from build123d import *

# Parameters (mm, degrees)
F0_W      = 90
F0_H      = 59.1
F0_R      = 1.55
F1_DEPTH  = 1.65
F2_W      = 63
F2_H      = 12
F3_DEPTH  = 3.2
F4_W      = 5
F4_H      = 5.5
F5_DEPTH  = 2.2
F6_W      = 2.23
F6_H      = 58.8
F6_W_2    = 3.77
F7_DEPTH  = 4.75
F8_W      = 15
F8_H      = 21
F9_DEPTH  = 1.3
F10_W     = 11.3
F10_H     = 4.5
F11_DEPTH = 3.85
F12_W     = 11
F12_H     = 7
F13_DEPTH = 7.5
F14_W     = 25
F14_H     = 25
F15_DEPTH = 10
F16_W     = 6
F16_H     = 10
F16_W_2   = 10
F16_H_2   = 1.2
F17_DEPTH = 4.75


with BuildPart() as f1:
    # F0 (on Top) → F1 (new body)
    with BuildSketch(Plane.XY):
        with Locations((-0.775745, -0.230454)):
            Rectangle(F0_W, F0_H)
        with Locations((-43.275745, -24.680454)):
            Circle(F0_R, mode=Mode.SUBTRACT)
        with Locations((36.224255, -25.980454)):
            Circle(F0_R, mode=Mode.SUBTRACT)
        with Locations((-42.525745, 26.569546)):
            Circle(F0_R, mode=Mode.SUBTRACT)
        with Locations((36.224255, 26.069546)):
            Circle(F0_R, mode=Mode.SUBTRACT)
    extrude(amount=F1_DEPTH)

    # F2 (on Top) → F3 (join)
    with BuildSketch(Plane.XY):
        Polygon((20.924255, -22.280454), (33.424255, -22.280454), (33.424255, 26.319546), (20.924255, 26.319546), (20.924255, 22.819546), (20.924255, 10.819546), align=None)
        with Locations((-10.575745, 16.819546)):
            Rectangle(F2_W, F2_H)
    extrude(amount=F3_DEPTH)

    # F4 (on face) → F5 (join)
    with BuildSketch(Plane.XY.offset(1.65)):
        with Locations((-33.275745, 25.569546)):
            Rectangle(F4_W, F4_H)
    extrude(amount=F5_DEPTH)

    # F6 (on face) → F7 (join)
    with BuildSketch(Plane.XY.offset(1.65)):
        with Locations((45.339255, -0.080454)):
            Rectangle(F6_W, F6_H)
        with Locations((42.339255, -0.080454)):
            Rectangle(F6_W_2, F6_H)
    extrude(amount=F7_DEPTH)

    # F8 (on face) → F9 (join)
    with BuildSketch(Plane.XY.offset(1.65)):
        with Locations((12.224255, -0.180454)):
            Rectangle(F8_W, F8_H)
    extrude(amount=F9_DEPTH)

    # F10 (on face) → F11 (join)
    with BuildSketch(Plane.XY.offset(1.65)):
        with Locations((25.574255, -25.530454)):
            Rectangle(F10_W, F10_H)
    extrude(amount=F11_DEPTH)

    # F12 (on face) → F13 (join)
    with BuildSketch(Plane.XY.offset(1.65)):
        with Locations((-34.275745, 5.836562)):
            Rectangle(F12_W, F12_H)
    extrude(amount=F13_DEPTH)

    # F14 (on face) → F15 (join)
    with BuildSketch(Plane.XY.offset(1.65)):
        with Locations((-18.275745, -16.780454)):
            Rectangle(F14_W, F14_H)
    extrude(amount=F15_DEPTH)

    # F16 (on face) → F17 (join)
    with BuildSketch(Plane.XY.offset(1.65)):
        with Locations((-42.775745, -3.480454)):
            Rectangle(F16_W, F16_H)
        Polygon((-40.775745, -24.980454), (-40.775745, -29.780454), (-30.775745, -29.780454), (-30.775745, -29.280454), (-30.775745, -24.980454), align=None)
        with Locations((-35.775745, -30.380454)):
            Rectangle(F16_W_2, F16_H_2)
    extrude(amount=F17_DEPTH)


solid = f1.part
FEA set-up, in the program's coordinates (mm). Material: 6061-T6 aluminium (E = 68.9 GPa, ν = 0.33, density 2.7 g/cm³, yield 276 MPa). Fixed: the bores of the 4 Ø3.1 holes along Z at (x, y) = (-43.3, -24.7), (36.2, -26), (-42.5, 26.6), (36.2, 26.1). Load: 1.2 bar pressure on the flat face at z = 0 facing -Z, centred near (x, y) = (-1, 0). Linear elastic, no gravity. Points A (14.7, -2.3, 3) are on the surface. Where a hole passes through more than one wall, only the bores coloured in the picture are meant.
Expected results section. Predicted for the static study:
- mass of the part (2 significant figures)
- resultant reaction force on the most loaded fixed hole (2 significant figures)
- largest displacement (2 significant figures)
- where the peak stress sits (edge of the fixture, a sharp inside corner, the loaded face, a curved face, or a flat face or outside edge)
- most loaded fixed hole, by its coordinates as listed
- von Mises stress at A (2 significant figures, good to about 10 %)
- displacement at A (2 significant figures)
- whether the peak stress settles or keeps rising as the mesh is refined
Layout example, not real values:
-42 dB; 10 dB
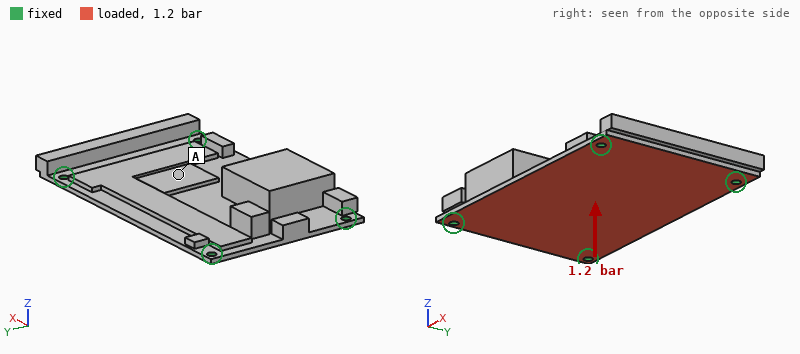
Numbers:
56 g; 340 N; 0.35 mm; edge of the fixture; (36.2, 26.1); 20 MPa; 0.25 mm; keeps rising
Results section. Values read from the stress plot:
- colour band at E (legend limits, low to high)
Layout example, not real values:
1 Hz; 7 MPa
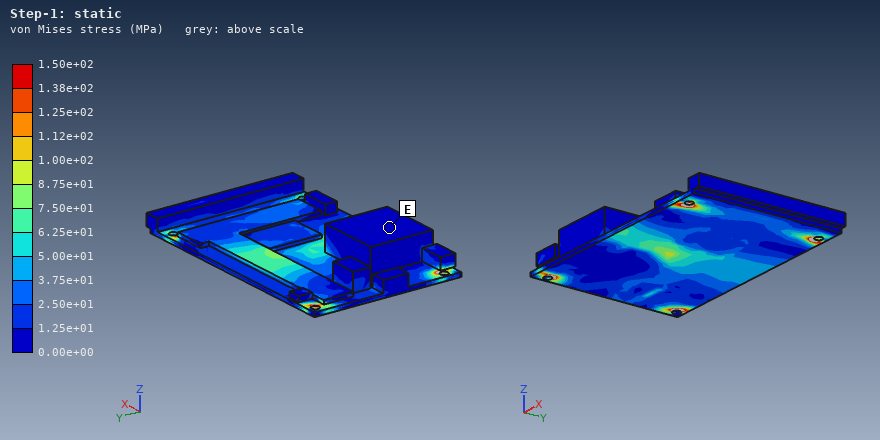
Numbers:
0.00e+00 to 1.25e+01 MPa
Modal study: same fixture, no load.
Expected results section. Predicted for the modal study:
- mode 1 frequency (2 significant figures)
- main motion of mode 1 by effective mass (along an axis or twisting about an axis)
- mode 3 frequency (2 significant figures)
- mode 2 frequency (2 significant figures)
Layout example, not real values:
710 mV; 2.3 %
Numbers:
1100 Hz; along Z; 3100 Hz; 2100 Hz
